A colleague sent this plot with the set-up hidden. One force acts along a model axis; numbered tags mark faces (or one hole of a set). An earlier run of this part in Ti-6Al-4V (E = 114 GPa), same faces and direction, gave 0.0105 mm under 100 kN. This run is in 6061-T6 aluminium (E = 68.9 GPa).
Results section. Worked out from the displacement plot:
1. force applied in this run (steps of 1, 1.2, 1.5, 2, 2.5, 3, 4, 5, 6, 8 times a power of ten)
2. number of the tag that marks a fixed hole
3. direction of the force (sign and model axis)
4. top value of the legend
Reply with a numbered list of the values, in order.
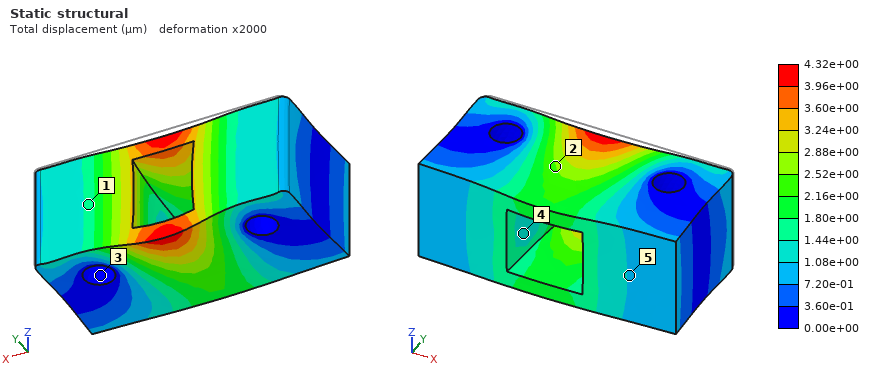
1. 25 kN
2. 3
3. -Y
4. 4.32e+00 µm
